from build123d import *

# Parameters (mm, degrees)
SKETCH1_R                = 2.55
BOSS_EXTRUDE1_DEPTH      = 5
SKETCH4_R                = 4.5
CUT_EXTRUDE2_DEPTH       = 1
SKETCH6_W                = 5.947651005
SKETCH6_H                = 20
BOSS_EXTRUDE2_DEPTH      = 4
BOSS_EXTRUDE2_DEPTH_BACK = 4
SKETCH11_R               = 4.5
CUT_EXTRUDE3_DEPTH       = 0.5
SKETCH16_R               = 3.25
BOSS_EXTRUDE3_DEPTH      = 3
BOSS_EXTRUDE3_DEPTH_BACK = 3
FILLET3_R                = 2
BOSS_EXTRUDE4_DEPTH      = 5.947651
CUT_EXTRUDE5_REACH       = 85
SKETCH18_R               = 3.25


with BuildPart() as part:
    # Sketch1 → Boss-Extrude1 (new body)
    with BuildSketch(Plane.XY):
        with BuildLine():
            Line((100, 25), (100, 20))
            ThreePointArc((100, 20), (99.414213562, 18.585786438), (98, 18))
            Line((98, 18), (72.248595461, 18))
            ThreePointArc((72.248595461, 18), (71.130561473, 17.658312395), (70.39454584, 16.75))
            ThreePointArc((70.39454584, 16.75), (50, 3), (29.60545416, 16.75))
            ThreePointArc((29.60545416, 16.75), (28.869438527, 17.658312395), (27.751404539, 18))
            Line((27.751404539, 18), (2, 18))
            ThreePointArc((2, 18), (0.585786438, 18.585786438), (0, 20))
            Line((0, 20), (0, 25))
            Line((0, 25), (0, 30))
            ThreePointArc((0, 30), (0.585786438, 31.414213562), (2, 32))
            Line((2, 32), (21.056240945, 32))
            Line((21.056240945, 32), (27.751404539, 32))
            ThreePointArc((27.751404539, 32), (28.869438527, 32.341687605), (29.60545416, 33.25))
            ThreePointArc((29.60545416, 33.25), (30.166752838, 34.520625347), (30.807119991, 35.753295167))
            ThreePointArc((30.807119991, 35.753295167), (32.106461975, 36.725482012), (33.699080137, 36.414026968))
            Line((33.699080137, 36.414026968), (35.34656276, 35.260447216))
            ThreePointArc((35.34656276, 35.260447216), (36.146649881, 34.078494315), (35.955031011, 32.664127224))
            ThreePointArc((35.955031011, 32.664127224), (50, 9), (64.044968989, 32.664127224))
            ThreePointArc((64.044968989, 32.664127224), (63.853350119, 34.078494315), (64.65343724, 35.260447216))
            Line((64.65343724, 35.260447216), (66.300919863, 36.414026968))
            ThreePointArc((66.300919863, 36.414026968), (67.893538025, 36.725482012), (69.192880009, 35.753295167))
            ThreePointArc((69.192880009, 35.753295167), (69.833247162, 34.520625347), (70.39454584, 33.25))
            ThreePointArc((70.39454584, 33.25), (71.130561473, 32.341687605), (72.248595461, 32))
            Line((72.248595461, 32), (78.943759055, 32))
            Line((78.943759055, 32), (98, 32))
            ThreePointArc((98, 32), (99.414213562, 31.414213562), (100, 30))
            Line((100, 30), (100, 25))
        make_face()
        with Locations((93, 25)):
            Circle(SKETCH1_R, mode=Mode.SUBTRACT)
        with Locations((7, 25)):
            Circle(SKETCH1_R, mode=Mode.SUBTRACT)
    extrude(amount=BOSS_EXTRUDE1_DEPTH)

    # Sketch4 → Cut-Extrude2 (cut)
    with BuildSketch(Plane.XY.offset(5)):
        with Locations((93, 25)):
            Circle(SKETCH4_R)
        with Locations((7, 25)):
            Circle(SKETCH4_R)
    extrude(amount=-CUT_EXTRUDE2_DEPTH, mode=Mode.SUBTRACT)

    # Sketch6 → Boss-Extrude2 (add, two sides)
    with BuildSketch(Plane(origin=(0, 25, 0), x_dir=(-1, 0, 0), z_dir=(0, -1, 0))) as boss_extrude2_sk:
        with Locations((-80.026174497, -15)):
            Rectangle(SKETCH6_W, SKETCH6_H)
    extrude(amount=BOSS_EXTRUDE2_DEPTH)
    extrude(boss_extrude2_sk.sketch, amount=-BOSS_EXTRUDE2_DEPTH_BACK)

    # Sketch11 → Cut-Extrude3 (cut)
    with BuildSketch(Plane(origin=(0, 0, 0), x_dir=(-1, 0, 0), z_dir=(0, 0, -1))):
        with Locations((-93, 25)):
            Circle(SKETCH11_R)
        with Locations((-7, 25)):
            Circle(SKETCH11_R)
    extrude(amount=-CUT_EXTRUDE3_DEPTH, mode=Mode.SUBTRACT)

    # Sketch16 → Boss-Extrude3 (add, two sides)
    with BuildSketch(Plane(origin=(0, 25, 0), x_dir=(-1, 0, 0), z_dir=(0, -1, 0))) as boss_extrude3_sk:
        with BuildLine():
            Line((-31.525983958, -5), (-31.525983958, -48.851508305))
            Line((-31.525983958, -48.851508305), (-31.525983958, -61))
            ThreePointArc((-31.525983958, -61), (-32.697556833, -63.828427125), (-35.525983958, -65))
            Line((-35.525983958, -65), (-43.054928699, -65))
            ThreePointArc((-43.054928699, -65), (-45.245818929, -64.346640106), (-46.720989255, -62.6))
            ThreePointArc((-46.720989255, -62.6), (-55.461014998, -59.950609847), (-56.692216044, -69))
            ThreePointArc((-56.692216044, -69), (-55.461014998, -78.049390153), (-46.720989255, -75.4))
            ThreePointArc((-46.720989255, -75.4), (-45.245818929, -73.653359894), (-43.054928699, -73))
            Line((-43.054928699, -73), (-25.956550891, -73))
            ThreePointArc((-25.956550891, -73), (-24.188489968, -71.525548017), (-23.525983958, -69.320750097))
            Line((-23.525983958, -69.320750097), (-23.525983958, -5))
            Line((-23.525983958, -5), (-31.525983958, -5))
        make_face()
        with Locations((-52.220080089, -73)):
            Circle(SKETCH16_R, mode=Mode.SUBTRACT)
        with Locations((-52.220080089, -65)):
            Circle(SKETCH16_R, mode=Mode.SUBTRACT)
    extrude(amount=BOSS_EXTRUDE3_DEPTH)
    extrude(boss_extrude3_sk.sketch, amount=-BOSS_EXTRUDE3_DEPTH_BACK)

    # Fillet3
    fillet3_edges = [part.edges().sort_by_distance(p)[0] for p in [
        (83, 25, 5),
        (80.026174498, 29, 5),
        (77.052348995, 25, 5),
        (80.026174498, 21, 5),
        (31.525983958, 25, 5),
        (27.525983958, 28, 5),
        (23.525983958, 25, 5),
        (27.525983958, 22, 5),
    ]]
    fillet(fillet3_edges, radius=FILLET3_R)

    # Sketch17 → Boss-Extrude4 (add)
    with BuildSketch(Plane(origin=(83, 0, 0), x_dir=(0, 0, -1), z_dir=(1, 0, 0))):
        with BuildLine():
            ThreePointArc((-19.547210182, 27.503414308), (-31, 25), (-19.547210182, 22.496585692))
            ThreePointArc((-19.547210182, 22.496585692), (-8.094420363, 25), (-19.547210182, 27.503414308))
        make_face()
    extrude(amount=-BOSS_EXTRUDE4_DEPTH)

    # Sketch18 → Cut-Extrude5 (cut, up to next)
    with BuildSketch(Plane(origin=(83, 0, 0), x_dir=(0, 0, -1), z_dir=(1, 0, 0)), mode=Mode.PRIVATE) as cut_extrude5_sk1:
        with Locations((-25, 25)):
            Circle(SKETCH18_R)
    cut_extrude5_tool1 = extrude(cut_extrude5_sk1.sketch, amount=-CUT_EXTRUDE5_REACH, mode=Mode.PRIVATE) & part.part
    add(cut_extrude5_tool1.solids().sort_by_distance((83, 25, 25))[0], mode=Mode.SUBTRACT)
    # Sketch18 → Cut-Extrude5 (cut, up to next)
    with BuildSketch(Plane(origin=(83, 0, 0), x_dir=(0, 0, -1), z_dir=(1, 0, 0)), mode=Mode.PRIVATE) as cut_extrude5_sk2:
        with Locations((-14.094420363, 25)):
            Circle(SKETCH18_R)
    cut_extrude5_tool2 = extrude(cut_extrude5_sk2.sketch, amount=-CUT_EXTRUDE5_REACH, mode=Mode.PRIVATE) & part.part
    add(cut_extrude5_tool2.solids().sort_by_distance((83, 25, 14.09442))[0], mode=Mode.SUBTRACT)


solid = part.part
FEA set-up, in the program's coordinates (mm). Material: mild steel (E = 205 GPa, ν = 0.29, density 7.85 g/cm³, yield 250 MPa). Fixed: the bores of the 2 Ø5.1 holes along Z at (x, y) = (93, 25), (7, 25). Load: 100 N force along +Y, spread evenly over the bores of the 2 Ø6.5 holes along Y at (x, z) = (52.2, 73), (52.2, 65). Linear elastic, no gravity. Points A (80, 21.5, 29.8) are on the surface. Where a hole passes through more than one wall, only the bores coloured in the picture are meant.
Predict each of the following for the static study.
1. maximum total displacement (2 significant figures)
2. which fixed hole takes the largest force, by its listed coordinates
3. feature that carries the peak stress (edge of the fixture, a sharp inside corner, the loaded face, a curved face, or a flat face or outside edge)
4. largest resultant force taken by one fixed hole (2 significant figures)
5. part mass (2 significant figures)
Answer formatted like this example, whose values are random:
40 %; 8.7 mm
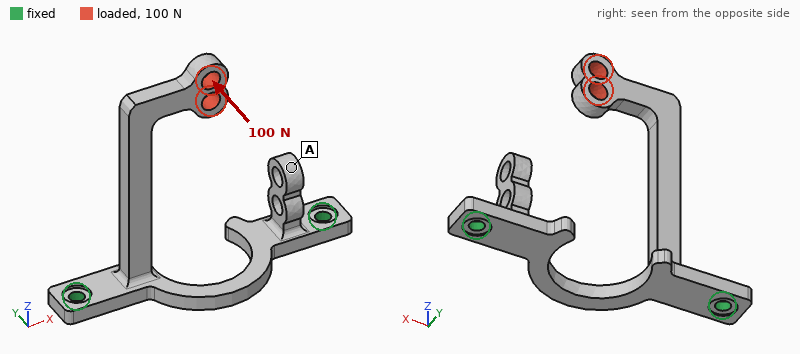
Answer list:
0.78 mm; (7, 25); a curved face; 92 N; 95 g
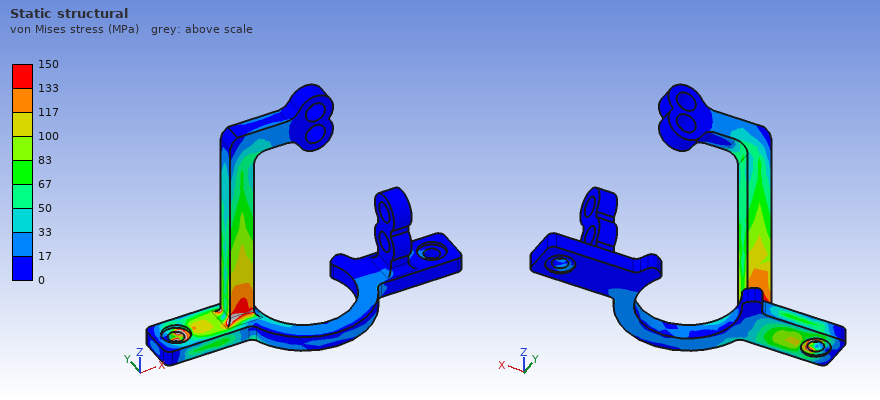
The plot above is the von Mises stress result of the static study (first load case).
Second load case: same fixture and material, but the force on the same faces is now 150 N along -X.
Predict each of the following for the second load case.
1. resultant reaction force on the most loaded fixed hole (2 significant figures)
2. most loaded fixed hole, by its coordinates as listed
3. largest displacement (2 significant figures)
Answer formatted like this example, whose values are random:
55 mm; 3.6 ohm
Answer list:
170 N; (7, 25); 0.69 mm
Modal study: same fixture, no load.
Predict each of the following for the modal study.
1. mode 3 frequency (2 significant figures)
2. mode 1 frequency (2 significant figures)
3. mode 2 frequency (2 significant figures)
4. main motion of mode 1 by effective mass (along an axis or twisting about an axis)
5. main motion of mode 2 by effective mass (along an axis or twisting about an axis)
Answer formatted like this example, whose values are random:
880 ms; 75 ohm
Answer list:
2000 Hz; 480 Hz; 560 Hz; along Y; along X
